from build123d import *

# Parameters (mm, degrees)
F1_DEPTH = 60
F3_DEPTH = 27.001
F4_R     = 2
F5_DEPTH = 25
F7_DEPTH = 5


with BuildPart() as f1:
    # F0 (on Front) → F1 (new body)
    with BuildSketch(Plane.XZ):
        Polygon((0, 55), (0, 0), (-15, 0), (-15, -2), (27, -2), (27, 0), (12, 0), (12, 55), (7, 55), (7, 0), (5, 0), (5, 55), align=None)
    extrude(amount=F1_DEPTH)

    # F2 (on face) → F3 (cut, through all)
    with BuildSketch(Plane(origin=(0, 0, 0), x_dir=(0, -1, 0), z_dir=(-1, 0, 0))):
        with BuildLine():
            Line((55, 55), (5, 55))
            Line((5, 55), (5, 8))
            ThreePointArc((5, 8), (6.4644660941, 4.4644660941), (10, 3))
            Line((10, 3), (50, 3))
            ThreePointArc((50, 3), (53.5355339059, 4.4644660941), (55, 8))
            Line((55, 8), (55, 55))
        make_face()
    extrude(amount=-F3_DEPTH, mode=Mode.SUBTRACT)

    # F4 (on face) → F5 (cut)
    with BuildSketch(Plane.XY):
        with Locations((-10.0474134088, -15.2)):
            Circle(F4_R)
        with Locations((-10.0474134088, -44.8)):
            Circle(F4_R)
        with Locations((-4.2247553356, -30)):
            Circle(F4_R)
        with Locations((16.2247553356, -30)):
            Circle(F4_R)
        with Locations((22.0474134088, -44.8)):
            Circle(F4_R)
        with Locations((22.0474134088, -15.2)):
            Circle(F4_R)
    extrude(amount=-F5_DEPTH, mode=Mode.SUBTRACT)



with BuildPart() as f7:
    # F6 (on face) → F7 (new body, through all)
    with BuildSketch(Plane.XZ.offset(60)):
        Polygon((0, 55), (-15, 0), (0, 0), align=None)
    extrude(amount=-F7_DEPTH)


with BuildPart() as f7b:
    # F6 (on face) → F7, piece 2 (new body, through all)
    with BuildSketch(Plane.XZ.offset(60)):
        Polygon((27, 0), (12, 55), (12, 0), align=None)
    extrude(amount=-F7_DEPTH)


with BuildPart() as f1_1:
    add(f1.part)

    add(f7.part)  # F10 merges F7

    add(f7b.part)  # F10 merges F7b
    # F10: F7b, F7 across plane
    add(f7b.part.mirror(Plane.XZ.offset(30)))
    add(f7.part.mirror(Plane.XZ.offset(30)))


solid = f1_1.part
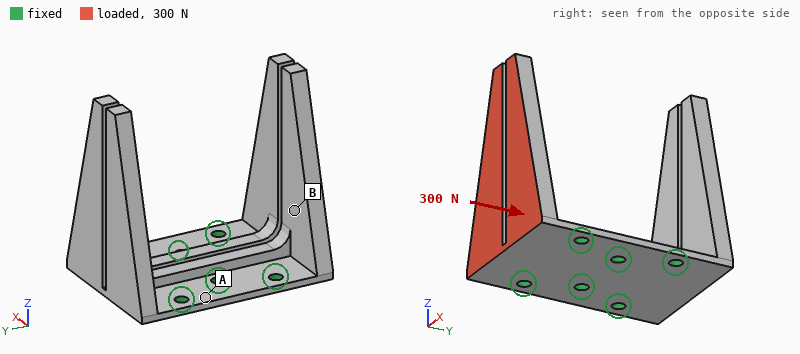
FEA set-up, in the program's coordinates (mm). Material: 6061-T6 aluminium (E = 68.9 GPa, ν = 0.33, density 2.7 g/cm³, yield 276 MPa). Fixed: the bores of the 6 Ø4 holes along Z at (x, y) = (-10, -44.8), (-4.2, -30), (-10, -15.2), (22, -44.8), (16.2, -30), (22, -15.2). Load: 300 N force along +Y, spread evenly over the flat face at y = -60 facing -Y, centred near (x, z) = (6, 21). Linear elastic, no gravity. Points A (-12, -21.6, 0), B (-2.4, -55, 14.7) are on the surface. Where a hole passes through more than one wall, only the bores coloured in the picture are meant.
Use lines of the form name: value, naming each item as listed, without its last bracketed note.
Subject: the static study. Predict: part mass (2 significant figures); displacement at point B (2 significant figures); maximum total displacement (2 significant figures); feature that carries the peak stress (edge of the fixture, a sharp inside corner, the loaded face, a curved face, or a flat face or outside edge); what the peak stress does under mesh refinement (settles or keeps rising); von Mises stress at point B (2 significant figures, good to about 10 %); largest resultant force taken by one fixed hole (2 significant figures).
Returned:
part mass: 55 g
displacement at point B: 0.16 mm
maximum total displacement: 0.66 mm
feature that carries the peak stress: edge of the fixture
what the peak stress does under mesh refinement: keeps rising
von Mises stress at point B: 22 MPa
largest resultant force taken by one fixed hole: 310 N
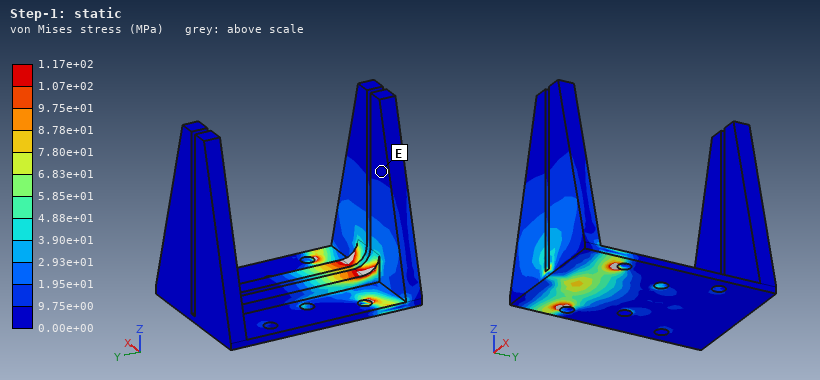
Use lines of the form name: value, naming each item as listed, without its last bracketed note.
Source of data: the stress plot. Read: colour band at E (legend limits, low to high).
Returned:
colour band at E: 0.00e+00 to 9.75e+00 MPa
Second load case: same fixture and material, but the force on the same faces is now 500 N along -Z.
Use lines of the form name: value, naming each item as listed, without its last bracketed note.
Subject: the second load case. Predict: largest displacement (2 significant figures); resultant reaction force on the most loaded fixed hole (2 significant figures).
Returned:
largest displacement: 0.57 mm
resultant reaction force on the most loaded fixed hole: 490 N
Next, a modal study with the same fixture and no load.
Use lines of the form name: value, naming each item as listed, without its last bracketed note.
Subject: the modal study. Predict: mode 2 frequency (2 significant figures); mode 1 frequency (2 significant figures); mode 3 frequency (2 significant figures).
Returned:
mode 2 frequency: 970 Hz
mode 1 frequency: 930 Hz
mode 3 frequency: 1500 Hz
